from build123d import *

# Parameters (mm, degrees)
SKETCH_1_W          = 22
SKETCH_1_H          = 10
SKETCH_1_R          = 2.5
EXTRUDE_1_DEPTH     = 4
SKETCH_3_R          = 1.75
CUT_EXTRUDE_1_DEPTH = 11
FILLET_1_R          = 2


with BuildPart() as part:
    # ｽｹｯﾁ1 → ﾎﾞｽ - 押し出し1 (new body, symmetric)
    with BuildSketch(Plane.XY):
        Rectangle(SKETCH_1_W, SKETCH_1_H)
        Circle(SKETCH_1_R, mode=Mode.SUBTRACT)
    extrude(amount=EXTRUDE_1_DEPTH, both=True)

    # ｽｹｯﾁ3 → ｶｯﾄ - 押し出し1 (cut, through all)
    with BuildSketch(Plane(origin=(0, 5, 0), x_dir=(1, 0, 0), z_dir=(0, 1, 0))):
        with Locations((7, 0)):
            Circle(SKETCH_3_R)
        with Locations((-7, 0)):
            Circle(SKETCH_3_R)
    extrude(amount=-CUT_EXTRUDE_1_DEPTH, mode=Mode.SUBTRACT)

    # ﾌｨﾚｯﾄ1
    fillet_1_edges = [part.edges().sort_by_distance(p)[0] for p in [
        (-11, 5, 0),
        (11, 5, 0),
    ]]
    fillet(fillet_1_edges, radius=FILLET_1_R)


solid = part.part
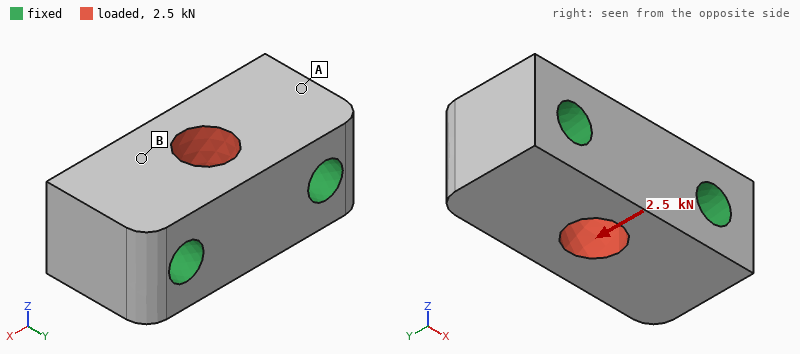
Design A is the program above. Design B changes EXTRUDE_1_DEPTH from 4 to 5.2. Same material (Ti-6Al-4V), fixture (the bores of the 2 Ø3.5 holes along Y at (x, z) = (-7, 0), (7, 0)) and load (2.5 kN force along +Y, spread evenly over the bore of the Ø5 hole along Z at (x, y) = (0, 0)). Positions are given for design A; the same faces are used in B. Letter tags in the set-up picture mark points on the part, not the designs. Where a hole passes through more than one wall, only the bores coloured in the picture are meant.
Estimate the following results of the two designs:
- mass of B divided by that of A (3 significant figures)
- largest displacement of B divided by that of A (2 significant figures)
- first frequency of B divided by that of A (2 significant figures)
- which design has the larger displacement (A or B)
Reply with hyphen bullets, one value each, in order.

- 1.34
- 0.88
- 0.92
- A
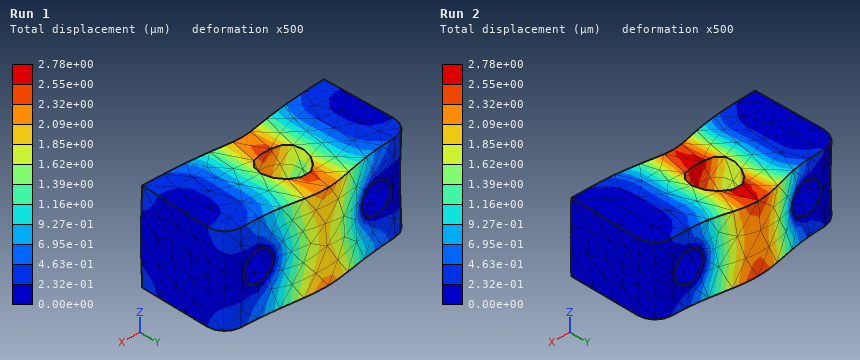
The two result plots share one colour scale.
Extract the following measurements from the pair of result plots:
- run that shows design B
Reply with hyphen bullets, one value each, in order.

- Run 1
